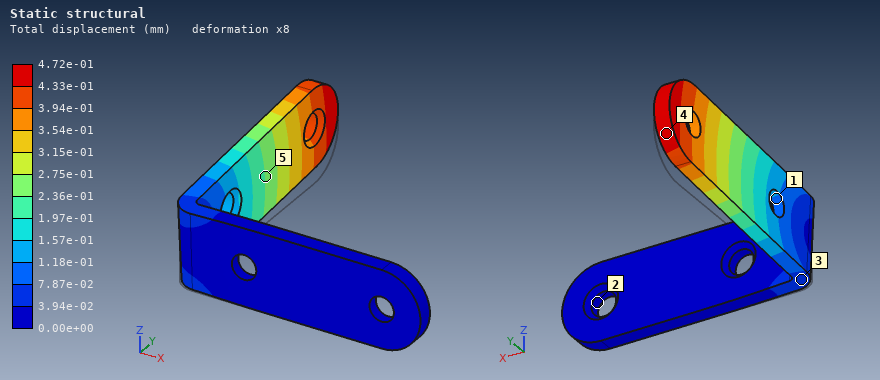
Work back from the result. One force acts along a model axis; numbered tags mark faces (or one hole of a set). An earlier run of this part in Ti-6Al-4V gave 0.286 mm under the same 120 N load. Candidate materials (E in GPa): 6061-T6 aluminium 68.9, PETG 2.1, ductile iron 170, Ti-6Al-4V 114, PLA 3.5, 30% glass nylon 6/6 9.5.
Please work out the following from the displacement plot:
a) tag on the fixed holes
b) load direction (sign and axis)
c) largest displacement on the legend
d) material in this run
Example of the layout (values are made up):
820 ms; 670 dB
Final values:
2; +Z; 4.72e-01 mm; 6061-T6 aluminium
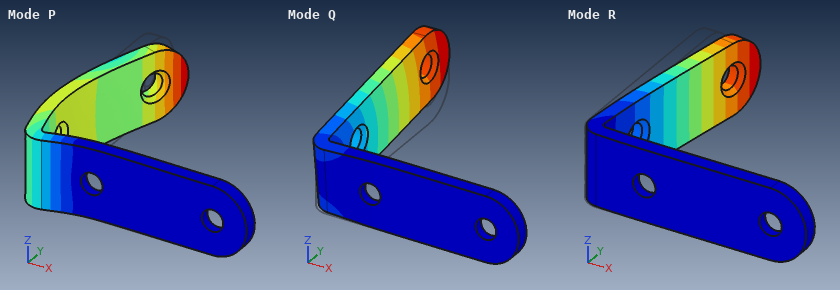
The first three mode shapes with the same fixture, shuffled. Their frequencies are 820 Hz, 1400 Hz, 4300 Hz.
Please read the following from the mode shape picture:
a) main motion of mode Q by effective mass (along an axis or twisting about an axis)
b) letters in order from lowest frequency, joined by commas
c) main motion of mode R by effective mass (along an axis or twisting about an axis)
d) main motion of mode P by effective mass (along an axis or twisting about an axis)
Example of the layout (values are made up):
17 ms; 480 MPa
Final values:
along Z; R, Q, P; along X; along Y
